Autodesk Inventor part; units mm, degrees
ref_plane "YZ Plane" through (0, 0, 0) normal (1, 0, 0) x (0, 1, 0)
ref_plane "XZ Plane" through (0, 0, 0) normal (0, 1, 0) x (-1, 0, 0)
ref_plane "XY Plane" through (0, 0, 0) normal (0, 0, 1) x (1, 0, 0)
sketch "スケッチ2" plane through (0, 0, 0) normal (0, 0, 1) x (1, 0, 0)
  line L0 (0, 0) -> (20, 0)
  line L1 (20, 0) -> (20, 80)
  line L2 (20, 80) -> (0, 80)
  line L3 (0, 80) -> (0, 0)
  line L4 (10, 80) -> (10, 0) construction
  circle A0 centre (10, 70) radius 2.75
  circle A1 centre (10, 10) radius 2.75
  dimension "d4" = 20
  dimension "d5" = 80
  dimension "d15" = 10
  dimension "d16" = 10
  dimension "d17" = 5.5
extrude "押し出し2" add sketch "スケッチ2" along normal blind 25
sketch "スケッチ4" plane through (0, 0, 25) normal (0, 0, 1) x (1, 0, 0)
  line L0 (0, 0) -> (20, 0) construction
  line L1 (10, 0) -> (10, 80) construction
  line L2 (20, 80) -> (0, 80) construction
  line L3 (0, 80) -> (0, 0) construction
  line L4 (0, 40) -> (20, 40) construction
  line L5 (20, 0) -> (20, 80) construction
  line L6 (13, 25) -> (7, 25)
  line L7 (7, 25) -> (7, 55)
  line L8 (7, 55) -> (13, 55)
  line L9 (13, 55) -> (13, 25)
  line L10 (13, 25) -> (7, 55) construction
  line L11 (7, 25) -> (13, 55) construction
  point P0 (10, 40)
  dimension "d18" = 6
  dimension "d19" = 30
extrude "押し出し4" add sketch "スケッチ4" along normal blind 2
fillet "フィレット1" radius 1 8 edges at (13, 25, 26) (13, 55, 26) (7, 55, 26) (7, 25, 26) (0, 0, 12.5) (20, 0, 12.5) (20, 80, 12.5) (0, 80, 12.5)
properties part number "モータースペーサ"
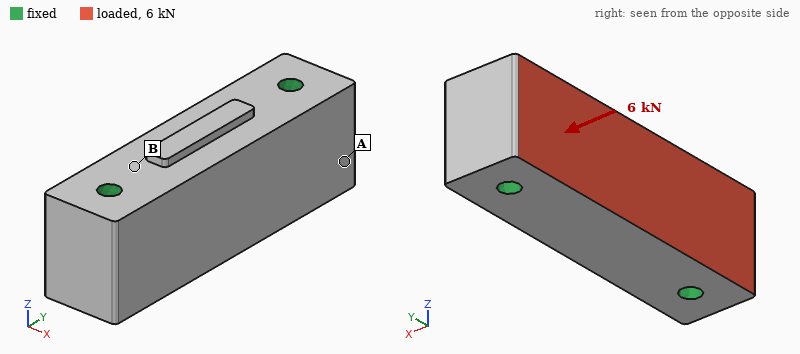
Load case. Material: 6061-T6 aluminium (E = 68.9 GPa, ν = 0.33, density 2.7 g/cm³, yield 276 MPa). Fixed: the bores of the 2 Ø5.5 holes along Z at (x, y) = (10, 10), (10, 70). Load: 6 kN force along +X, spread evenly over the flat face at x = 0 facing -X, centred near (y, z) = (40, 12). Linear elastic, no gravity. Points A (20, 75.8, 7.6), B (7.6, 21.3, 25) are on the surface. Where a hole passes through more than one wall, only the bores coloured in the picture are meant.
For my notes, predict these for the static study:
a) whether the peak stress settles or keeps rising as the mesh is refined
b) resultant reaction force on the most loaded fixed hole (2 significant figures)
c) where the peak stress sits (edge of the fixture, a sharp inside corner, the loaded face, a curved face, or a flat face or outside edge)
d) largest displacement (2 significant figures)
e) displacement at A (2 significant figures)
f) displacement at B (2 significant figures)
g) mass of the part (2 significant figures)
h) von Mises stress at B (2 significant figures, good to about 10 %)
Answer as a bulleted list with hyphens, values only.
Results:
- keeps rising
- 3.0 kN
- edge of the fixture
- 7.7 µm
- 1.6 µm
- 3.9 µm
- 110 g
- 8.1 MPa
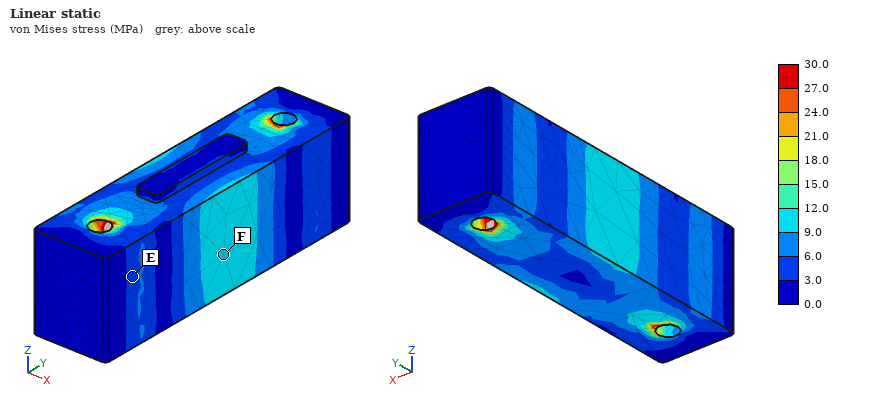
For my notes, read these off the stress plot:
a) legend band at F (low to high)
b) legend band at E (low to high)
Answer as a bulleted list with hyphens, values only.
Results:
- 9.0 to 12.0 MPa
- 3.0 to 6.0 MPa
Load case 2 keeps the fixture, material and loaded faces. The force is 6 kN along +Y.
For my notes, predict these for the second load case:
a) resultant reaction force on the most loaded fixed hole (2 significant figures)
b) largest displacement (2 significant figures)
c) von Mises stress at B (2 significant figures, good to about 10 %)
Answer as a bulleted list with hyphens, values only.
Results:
- 3.1 kN
- 2.6 µm
- 5.8 MPa
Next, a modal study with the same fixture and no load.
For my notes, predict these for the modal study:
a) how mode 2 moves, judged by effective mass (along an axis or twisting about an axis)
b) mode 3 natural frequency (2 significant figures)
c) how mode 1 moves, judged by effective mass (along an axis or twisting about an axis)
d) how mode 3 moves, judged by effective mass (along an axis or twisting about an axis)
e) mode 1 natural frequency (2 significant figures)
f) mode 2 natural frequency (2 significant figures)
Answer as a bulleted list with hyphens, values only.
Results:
- along Z
- 23 kHz
- along X
- twisting about Y
- 15 kHz
- 20 kHz
